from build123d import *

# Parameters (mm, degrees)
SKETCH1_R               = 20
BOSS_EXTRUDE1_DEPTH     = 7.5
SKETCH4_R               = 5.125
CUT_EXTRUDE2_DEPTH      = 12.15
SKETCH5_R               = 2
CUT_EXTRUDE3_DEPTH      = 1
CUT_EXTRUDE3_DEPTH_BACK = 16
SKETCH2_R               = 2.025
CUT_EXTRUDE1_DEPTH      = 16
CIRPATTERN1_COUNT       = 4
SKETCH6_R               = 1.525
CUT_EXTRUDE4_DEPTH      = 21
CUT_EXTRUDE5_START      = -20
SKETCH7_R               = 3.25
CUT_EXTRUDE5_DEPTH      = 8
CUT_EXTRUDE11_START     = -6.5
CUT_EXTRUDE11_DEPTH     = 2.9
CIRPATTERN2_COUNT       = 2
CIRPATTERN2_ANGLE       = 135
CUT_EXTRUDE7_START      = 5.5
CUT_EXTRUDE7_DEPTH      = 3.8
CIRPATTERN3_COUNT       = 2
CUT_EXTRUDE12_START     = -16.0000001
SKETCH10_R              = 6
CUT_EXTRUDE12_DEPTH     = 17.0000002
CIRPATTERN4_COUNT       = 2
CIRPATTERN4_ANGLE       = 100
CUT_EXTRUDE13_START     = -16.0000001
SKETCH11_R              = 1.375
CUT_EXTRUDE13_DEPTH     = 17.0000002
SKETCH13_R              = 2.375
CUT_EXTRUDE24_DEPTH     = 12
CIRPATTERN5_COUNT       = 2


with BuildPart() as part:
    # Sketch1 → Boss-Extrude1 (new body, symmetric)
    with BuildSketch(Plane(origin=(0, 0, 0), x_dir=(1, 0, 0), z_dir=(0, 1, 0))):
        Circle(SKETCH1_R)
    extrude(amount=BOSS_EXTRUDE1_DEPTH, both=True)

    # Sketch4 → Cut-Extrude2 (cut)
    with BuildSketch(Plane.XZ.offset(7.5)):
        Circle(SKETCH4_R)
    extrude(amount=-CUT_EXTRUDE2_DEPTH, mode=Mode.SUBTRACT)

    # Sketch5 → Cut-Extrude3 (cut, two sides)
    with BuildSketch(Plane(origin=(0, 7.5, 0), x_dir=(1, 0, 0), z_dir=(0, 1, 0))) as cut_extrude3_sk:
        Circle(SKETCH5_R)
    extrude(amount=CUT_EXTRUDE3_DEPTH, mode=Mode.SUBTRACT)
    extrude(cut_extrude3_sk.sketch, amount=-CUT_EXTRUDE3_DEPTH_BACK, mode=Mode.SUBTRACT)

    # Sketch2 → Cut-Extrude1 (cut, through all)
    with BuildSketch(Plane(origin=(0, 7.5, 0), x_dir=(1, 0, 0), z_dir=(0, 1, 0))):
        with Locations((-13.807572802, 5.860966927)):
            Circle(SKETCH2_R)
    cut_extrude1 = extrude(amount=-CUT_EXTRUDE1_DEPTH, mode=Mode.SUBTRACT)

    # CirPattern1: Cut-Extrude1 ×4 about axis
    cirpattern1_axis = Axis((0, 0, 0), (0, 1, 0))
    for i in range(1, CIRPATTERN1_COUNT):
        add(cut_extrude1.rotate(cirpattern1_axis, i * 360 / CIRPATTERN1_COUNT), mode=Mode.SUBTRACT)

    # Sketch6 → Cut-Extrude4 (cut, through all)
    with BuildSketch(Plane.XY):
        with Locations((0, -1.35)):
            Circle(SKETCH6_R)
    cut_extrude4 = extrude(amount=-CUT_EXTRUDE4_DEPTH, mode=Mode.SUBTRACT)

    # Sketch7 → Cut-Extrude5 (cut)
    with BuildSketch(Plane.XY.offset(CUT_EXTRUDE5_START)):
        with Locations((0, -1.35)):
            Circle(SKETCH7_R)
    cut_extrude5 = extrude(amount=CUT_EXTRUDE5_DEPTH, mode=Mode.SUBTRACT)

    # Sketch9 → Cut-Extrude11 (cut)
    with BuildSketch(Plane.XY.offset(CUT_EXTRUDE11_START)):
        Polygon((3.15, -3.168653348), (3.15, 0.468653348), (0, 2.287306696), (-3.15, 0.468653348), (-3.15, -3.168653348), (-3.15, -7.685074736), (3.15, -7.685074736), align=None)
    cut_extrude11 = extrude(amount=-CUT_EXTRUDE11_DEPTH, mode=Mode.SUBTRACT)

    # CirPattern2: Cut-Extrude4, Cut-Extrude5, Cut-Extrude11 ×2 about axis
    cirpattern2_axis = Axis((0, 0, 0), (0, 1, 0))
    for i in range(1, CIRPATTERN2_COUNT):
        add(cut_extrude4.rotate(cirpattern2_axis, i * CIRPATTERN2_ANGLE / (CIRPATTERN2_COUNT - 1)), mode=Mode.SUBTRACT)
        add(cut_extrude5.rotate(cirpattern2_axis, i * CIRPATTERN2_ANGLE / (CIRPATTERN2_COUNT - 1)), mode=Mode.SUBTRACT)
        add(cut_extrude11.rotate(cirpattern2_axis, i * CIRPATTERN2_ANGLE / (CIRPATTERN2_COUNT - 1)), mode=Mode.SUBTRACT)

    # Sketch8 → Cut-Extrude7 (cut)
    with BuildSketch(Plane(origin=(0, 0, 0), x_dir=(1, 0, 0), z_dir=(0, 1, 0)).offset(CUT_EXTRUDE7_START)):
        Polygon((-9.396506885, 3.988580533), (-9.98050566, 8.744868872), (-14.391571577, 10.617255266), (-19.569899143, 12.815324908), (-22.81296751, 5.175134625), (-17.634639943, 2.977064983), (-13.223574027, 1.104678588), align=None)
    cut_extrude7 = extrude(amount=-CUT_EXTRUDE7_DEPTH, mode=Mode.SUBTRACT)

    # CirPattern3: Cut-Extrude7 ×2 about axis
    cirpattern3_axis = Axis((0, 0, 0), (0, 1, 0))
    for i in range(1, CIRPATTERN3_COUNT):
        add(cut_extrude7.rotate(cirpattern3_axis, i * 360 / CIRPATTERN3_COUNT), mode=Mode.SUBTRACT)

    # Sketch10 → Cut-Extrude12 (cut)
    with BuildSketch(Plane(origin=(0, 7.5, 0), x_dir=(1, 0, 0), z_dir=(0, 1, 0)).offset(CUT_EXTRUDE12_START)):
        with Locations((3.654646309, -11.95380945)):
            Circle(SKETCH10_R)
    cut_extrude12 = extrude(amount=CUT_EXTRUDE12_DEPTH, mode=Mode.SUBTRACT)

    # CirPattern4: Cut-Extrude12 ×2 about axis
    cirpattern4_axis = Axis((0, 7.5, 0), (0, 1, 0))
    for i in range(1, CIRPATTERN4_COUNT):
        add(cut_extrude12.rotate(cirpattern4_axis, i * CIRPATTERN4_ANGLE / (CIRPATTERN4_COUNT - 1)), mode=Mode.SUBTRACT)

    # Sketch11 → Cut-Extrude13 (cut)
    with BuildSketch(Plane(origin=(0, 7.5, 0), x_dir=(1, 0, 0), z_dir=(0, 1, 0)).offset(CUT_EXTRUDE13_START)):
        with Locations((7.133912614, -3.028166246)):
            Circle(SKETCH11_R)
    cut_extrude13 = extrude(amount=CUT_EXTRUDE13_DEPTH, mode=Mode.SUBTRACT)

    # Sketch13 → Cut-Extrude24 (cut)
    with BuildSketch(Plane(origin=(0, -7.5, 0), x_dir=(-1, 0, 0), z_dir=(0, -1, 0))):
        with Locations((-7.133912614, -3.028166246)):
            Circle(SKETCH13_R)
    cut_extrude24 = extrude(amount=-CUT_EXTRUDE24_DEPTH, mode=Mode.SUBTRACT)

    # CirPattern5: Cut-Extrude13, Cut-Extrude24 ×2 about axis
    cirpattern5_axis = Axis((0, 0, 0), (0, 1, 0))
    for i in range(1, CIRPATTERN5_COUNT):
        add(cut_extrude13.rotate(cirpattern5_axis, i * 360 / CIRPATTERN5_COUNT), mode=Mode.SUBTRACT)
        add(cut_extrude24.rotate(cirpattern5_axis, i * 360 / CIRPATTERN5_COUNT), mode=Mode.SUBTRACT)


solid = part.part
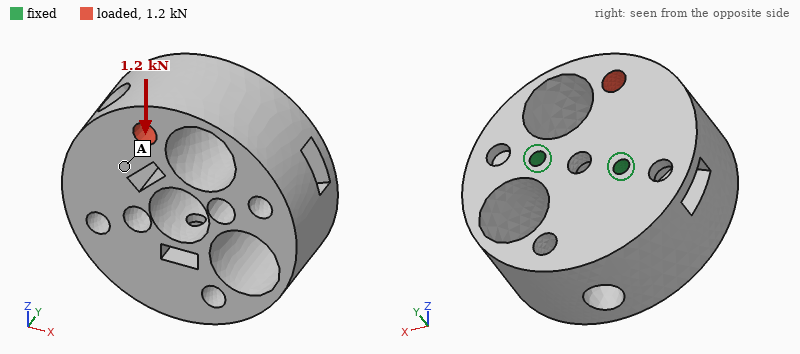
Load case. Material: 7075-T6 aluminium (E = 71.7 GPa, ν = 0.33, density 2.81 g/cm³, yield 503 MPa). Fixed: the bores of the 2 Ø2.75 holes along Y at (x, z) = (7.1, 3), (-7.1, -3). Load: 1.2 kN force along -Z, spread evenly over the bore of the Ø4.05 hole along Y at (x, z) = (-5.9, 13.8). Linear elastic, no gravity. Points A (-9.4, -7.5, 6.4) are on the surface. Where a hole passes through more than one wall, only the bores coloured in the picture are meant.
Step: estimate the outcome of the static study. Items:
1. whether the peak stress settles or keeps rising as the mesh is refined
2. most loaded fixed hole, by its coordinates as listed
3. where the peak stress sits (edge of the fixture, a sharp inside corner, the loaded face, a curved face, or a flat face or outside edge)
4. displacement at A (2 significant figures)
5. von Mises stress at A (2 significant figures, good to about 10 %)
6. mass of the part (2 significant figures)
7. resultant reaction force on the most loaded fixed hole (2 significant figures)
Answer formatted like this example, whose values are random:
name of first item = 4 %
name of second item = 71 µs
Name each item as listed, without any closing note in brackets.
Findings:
whether the peak stress settles or keeps rising as the mesh is refined = keeps rising
most loaded fixed hole, by its coordinates as listed = (-7.1, -3)
where the peak stress sits = edge of the fixture
displacement at A = 43 µm
von Mises stress at A = 17 MPa
mass of the part = 33 g
resultant reaction force on the most loaded fixed hole = 1.1 kN
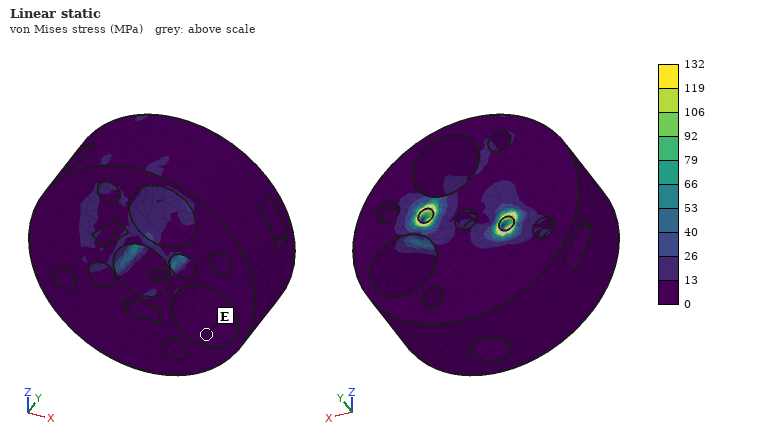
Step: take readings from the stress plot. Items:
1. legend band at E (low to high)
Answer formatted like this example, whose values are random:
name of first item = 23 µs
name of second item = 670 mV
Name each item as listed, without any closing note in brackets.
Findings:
legend band at E = 0 to 13 MPa
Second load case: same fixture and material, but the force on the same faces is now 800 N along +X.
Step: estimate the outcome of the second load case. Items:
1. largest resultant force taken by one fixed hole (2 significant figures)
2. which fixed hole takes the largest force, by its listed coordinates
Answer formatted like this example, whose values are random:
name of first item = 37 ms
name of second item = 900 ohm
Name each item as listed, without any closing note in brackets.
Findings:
largest resultant force taken by one fixed hole = 910 N
which fixed hole takes the largest force, by its listed coordinates = (7.1, 3)
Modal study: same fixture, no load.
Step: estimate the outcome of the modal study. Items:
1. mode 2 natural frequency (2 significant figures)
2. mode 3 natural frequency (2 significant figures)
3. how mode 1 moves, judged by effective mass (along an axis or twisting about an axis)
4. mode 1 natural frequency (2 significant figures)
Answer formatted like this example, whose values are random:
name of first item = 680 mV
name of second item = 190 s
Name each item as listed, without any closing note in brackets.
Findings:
mode 2 natural frequency = 10000 Hz
mode 3 natural frequency = 10 kHz
how mode 1 moves, judged by effective mass = along Z
mode 1 natural frequency = 3600 Hz
